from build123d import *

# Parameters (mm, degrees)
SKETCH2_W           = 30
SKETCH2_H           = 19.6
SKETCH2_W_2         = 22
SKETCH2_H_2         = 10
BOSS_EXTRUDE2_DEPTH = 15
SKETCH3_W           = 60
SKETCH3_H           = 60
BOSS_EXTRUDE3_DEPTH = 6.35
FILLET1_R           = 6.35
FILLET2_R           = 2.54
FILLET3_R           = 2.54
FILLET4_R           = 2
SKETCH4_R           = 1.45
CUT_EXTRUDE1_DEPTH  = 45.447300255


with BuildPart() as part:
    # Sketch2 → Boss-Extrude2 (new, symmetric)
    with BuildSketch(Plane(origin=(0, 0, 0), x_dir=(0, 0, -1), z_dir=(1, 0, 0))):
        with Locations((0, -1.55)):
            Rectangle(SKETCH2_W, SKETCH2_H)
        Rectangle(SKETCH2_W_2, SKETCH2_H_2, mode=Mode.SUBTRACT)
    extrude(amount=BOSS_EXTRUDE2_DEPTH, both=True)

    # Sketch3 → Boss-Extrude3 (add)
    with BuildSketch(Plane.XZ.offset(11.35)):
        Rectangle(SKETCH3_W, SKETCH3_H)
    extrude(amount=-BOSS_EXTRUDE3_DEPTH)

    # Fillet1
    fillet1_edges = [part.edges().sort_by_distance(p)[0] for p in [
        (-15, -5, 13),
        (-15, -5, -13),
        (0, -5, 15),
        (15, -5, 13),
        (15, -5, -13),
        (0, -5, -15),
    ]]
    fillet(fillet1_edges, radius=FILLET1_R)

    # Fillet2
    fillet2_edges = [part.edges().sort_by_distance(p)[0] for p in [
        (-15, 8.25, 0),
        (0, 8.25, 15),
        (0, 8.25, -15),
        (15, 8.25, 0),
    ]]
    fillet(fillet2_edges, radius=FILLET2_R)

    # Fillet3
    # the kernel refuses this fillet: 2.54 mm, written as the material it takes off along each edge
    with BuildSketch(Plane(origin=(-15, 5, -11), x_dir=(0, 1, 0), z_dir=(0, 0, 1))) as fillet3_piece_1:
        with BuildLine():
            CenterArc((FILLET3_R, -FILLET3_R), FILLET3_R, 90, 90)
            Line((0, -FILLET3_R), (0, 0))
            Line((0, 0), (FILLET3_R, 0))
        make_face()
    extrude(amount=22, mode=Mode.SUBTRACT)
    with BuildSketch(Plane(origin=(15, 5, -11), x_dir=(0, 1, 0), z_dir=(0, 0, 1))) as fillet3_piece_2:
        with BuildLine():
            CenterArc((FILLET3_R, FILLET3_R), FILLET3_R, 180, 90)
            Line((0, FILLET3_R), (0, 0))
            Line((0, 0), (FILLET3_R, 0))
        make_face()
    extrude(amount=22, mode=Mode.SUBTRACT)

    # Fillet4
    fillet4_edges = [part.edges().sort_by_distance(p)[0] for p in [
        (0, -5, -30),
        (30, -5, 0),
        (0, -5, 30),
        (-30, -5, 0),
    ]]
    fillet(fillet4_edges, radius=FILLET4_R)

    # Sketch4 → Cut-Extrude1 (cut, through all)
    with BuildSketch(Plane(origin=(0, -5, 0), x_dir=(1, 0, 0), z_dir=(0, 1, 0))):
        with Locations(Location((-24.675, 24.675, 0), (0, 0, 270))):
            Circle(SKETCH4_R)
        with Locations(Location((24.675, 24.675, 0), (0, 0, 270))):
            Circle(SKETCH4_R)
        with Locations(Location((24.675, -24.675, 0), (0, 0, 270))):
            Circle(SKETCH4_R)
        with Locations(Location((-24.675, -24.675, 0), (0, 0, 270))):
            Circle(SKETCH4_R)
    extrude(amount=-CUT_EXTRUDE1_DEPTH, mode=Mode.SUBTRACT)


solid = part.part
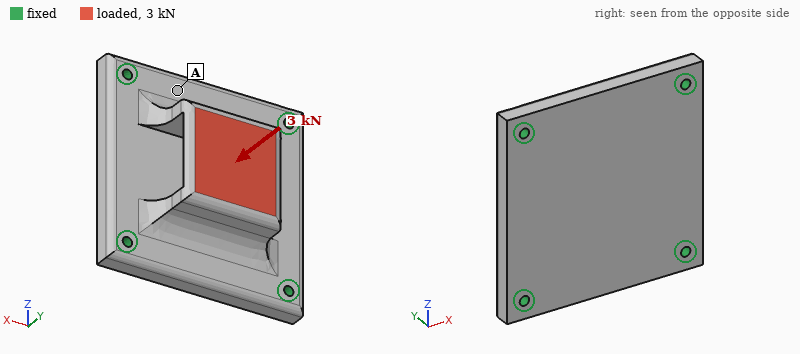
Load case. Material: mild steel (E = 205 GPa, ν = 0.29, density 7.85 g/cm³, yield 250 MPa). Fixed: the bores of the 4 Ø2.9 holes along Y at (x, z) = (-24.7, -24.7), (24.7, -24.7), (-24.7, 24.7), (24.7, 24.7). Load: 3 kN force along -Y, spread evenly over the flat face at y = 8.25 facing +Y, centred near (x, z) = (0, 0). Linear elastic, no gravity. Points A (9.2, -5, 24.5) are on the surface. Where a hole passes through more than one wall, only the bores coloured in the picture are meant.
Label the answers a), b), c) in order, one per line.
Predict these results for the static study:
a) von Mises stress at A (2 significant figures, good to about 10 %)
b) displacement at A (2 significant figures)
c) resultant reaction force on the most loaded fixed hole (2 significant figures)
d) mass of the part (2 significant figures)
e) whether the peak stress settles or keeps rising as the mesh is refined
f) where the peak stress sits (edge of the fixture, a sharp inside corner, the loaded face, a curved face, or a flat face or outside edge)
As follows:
a) 13 MPa
b) 4.8 µm
c) 810 N
d) 220 g
e) keeps rising
f) edge of the fixture
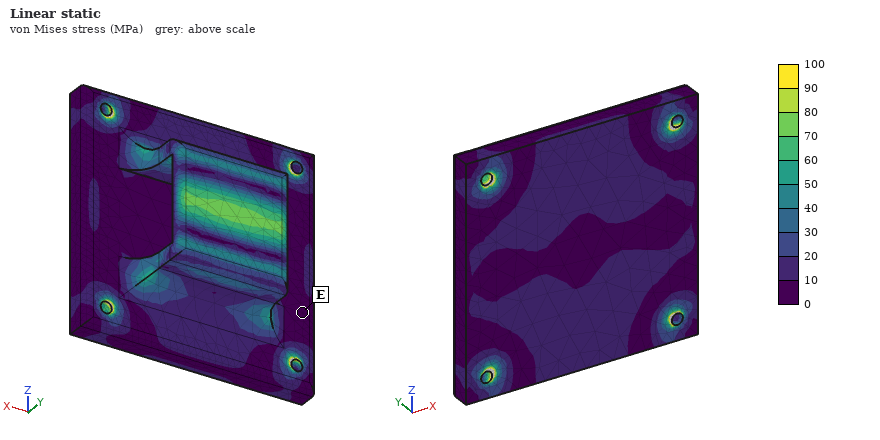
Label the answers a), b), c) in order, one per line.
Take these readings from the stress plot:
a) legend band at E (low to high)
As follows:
a) 0 to 10 MPa
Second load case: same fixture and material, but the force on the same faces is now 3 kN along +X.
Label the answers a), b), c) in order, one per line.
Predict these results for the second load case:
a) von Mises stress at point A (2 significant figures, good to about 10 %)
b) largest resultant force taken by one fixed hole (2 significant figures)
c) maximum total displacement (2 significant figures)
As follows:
a) 14 MPa
b) 990 N
c) 9.1 µm
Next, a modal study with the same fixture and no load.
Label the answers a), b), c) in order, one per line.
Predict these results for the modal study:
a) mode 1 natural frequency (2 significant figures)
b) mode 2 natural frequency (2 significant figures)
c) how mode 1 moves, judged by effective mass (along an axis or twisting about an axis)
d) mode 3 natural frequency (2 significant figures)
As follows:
a) 8200 Hz
b) 12 kHz
c) along Y
d) 13 kHz
